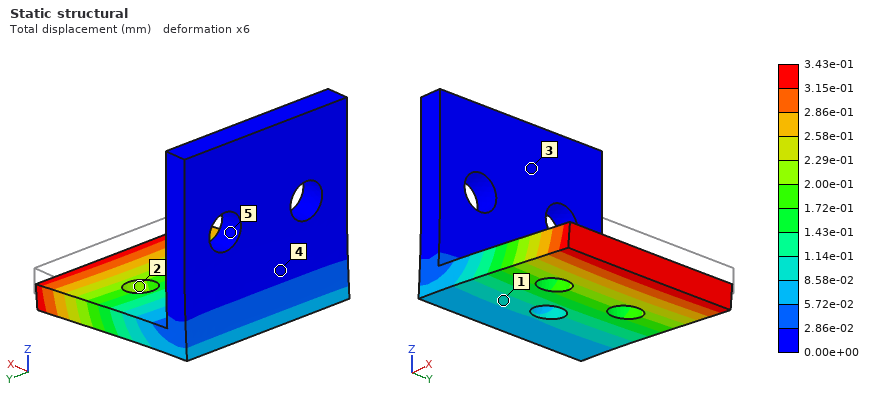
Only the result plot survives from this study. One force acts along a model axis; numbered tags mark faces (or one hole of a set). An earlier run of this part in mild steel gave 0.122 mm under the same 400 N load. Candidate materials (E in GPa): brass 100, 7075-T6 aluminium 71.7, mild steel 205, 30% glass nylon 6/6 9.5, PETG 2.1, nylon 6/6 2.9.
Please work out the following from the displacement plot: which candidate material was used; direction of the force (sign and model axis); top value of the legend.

7075-T6 aluminium
-Z
3.43e-01 mm
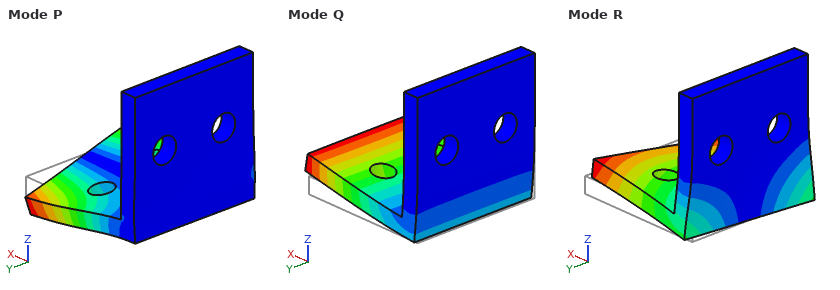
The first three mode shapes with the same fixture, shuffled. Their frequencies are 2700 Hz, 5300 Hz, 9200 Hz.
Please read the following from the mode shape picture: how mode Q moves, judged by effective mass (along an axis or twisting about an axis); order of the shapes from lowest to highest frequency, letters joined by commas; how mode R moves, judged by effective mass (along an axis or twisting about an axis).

along Z
Q, R, P
along Y
